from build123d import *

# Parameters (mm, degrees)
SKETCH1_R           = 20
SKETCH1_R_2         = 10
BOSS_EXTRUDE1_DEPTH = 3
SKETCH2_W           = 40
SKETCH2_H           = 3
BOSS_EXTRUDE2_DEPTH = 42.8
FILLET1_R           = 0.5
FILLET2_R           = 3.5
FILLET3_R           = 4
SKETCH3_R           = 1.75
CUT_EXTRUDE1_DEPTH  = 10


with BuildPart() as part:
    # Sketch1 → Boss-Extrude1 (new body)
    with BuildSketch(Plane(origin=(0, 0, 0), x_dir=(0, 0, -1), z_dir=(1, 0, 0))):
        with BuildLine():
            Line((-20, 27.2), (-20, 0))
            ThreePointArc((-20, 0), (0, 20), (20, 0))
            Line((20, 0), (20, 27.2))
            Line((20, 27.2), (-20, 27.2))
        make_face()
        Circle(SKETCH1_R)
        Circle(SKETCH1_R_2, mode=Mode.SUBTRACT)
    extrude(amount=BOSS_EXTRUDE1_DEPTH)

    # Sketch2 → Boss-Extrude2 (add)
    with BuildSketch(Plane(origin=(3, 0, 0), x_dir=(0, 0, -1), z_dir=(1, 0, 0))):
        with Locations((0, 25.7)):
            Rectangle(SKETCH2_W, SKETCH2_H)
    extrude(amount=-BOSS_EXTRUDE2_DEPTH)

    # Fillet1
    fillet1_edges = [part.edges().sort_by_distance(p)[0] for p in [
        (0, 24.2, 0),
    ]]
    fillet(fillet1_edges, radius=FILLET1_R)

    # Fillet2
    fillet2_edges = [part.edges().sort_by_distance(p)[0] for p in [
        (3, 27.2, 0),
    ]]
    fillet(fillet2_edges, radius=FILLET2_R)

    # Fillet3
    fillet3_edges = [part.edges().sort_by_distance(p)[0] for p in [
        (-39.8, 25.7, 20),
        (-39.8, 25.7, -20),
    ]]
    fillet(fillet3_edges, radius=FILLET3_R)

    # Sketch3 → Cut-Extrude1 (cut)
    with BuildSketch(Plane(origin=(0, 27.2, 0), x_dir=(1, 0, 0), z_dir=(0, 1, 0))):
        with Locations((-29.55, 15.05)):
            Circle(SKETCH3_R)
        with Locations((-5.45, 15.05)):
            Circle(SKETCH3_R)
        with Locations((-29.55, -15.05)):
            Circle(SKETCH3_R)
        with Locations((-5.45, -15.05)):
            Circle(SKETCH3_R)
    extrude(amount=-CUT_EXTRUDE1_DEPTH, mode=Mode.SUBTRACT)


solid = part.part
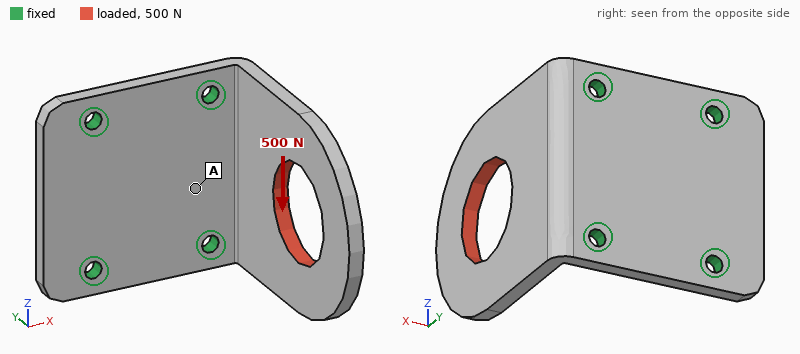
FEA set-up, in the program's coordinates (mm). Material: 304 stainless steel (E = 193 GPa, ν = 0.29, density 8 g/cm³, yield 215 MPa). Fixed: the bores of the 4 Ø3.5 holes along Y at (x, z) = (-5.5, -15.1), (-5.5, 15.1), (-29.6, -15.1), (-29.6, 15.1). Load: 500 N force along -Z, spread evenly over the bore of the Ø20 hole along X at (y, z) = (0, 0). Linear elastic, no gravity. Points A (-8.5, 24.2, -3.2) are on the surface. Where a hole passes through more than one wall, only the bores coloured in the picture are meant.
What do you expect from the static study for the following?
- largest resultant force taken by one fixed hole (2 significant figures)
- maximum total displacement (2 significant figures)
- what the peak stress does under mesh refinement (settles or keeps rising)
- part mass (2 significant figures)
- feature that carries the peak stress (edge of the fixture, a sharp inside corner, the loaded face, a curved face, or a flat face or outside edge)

500 N
24 µm
keeps rising
70 g
edge of the fixture
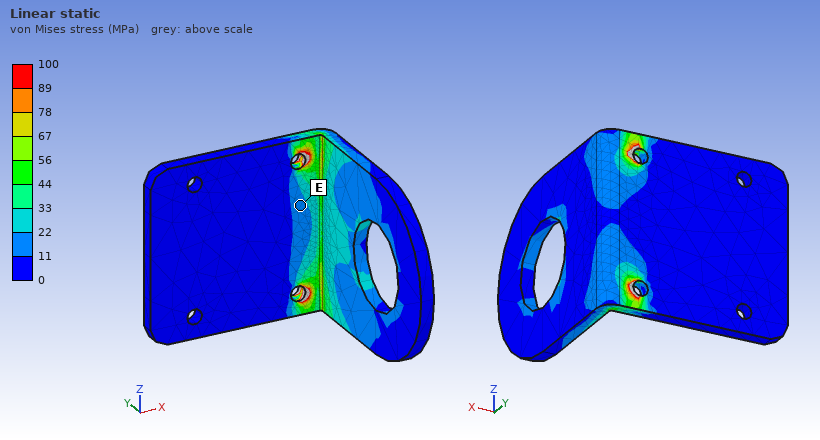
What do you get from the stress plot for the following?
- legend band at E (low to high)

11 to 22 MPa
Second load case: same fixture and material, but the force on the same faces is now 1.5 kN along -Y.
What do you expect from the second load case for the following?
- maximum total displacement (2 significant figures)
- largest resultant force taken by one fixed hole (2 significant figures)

0.10 mm
790 N
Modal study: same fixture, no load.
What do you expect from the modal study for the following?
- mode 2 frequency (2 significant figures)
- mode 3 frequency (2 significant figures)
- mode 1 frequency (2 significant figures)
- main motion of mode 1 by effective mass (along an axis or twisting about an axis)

3200 Hz
5700 Hz
1100 Hz
along X
